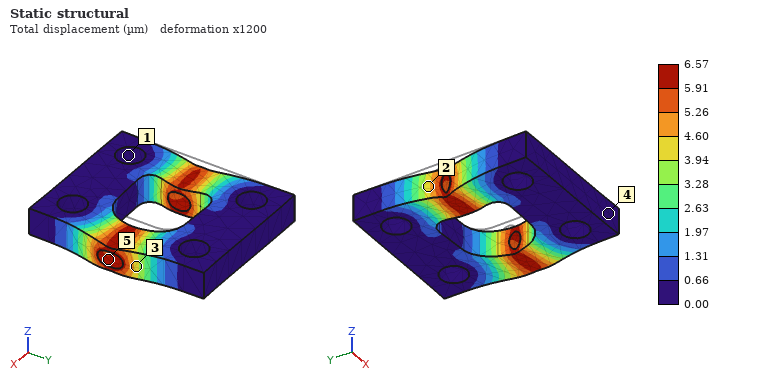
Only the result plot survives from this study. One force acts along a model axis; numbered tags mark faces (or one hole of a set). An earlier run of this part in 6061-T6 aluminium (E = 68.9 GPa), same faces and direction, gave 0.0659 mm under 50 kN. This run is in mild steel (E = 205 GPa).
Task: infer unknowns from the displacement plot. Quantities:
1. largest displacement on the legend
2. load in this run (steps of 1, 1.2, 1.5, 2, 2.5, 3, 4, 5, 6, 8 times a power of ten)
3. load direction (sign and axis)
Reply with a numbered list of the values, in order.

1. 6.57 µm
2. 15 kN
3. +X
